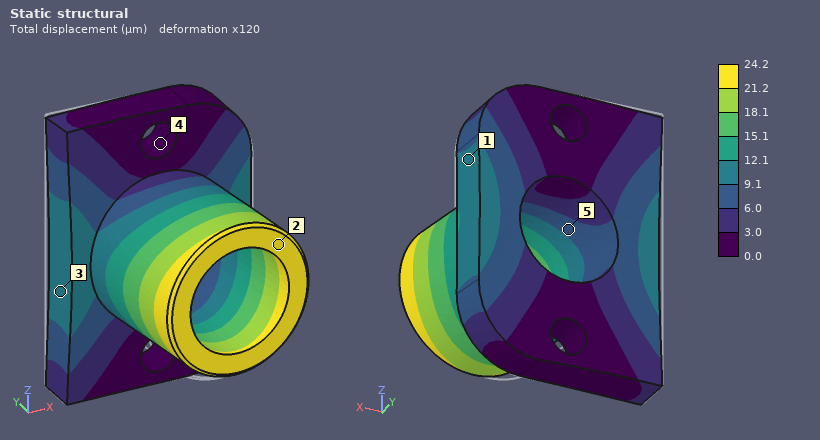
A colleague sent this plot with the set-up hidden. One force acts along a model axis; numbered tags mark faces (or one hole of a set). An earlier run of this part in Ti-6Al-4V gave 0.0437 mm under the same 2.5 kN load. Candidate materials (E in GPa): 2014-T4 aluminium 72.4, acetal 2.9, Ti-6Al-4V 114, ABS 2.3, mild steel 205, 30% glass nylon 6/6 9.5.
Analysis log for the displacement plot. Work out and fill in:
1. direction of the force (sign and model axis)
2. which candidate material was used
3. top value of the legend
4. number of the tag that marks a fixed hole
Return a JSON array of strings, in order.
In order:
["+X", "mild steel", "24.2 µm", "4"]
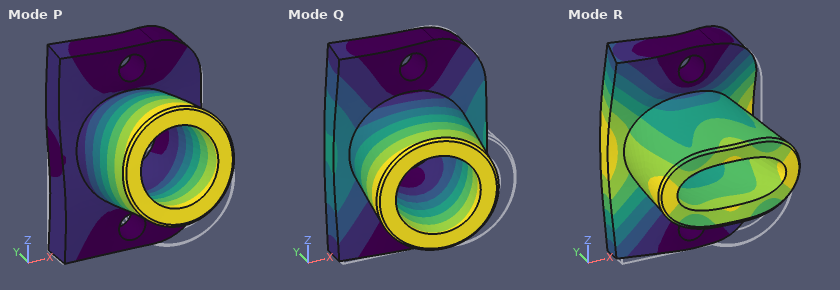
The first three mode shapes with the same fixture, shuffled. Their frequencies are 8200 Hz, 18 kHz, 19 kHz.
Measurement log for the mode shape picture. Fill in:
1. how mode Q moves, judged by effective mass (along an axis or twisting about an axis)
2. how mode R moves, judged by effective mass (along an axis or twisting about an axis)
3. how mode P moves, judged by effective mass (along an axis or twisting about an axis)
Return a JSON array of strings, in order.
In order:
["along X", "along Y", "along Z"]
